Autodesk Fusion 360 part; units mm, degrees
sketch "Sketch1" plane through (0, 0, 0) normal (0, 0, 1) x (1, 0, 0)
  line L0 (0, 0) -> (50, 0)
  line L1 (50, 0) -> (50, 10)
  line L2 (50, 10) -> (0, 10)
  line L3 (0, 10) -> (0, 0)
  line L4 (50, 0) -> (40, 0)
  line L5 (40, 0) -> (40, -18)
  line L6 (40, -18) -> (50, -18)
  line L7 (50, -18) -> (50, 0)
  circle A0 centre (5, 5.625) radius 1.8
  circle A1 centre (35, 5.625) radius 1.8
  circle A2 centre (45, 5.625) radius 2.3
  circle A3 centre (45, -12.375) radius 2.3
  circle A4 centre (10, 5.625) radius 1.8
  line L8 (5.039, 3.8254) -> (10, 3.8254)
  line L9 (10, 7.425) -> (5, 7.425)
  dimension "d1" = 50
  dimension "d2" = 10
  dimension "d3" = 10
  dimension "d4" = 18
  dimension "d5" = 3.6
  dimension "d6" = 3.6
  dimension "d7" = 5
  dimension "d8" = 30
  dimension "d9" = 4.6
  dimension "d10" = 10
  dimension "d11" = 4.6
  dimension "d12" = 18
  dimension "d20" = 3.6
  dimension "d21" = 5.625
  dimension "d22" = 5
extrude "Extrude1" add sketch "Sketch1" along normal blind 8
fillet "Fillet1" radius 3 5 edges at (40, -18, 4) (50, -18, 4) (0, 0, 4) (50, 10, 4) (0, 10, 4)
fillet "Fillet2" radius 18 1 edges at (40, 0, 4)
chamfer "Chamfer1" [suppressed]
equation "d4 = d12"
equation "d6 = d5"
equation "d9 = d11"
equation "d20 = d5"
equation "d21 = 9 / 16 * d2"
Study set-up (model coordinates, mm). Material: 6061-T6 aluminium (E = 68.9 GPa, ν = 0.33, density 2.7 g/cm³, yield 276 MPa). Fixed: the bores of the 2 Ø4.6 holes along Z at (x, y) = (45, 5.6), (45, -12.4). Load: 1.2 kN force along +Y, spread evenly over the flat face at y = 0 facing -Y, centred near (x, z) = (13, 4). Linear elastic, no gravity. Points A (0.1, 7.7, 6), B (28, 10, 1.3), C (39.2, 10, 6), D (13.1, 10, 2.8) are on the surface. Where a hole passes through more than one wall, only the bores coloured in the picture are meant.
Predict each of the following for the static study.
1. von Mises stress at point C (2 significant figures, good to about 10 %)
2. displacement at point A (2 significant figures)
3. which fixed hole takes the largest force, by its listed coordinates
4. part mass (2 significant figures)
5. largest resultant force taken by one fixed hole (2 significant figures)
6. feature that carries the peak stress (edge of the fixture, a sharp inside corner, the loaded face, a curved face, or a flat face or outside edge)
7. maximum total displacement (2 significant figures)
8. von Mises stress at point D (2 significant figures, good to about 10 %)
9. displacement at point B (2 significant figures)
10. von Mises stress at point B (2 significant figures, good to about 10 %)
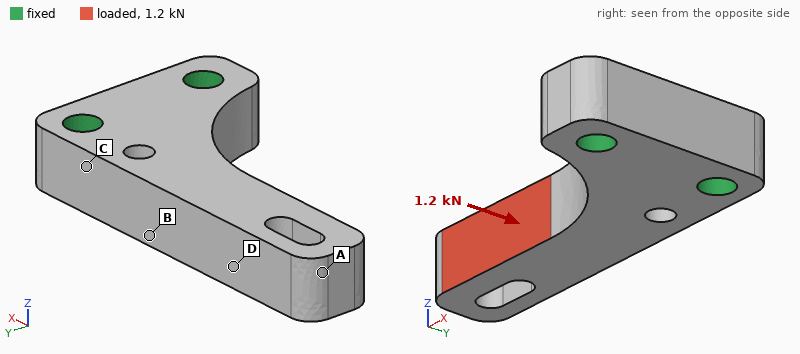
100 MPa
0.22 mm
(45, -12.4)
14 g
2.3 kN
a curved face
0.22 mm
27 MPa
0.039 mm
120 MPa
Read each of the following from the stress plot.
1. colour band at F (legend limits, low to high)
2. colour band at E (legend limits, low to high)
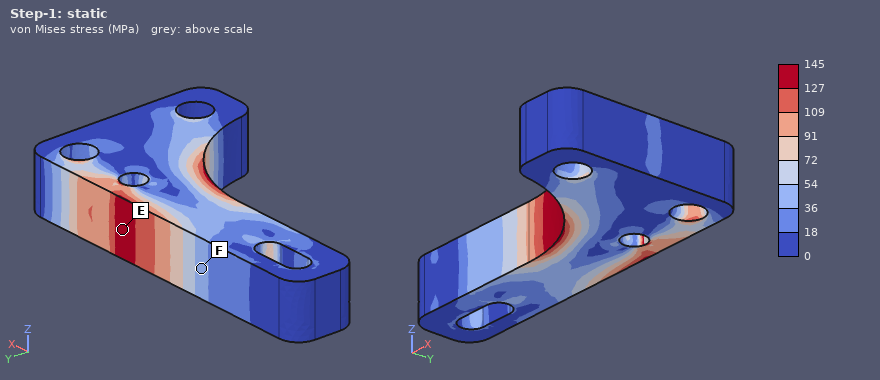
36 to 54 MPa
127 to 145 MPa
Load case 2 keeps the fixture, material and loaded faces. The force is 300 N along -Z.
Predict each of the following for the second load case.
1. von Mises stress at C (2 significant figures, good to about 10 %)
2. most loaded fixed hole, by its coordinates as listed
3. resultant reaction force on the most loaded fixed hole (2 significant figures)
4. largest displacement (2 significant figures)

29 MPa
(45, 5.6)
220 N
0.15 mm
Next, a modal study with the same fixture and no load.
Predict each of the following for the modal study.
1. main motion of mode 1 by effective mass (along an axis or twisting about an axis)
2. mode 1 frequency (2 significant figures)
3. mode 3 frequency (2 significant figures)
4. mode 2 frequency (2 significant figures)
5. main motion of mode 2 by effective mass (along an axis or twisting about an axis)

along Z
4000 Hz
18 kHz
6600 Hz
along Y
